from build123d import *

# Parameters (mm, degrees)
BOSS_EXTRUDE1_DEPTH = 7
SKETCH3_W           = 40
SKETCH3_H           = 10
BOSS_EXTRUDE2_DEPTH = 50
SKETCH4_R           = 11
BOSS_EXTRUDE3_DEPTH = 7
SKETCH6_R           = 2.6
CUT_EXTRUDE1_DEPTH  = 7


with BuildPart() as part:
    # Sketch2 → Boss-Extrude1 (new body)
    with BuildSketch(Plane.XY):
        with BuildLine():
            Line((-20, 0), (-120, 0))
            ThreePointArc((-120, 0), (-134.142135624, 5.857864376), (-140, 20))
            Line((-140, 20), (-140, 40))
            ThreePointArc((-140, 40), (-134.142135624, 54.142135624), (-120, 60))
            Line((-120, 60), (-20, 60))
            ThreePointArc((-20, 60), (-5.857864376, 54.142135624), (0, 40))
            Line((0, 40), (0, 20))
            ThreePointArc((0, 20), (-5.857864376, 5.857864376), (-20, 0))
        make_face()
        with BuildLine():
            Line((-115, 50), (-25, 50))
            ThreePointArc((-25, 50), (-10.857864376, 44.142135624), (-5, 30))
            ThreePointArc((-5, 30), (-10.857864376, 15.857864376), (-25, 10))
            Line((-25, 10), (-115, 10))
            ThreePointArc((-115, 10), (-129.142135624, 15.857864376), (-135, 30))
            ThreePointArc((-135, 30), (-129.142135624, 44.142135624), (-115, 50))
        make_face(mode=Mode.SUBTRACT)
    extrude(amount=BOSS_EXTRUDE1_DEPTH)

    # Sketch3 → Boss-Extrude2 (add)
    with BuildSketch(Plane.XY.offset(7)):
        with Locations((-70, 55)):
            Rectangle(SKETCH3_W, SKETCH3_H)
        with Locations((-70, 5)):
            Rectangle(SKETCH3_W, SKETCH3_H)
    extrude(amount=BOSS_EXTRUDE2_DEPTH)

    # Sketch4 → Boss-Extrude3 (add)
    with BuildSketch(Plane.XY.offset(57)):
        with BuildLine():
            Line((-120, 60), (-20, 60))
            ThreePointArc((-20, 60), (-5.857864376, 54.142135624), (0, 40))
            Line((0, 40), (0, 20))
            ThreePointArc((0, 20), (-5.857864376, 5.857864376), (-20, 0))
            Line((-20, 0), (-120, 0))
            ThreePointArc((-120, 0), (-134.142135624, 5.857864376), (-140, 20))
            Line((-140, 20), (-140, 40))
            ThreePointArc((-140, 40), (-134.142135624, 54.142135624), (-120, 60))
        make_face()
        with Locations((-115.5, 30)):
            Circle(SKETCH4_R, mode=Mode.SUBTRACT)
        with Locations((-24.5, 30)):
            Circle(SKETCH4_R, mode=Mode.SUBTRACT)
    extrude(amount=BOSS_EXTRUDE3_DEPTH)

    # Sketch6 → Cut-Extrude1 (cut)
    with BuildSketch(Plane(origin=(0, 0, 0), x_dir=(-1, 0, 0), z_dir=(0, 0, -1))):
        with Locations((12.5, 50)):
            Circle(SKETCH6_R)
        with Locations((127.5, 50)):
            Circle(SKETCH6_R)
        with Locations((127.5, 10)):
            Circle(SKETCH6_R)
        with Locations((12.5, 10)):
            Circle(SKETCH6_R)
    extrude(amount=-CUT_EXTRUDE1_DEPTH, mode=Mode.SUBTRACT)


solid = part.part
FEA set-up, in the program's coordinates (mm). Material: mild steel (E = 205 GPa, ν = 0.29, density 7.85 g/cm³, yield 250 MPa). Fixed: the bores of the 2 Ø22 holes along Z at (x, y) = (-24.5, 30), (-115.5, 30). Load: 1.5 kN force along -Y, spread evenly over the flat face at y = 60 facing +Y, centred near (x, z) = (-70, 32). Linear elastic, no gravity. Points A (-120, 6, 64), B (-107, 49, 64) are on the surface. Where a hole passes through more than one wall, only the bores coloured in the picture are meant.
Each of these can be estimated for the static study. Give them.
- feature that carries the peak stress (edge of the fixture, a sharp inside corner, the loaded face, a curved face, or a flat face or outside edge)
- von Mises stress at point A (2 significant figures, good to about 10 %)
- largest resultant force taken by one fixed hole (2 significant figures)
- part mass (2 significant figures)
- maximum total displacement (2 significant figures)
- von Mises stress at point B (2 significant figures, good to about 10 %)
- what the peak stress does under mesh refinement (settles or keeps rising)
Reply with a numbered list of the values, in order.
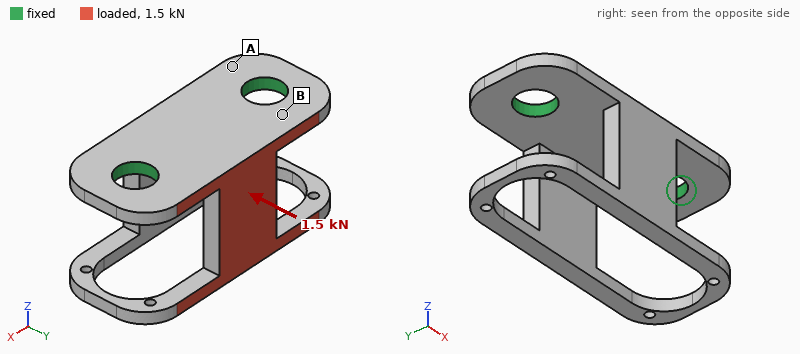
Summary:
1. a sharp inside corner
2. 11 MPa
3. 750 N
4. 890 g
5. 0.12 mm
6. 29 MPa
7. keeps rising
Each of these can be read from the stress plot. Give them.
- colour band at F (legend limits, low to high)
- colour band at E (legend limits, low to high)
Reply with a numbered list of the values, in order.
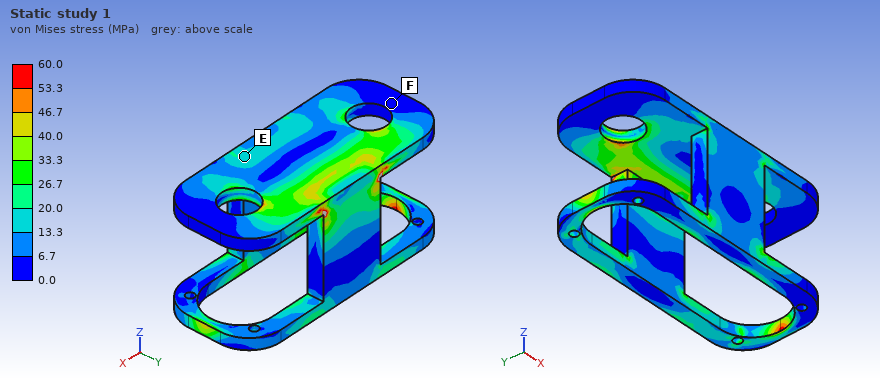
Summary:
1. 0.0 to 6.7 MPa
2. 13.3 to 20.0 MPa
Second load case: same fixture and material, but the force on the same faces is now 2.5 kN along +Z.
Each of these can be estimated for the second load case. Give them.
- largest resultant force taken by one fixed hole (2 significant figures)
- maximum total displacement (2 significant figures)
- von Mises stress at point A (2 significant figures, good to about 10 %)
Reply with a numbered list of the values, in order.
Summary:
1. 1.3 kN
2. 97 µm
3. 9.3 MPa
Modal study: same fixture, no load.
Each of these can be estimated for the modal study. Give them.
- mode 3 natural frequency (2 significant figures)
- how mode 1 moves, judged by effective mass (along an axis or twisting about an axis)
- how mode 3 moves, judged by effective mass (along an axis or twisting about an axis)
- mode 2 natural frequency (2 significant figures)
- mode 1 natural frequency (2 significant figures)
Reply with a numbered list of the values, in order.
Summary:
1. 1600 Hz
2. along Y
3. along Z
4. 1400 Hz
5. 910 Hz
